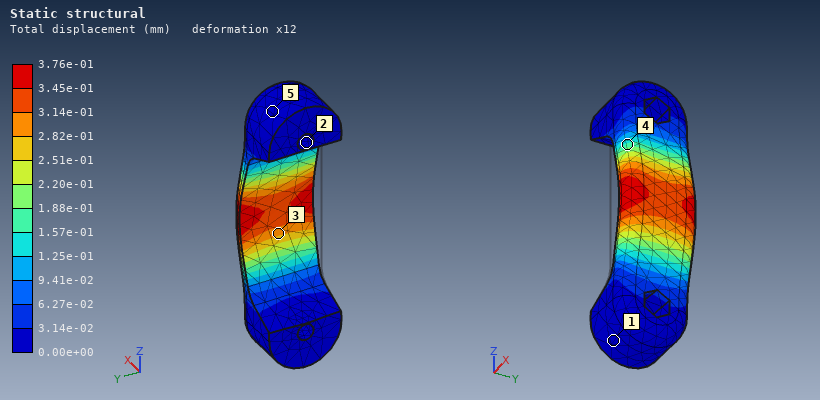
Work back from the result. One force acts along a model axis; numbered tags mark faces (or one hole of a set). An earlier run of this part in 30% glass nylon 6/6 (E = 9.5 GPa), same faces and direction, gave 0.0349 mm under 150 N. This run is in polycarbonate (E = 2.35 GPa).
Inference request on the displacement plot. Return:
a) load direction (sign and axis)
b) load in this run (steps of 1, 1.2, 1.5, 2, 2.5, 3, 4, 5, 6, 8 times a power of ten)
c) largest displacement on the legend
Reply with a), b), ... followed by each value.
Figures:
a) +X
b) 400 N
c) 3.76e-01 mm
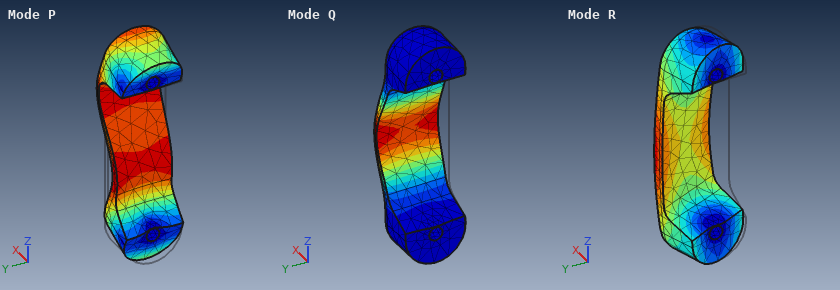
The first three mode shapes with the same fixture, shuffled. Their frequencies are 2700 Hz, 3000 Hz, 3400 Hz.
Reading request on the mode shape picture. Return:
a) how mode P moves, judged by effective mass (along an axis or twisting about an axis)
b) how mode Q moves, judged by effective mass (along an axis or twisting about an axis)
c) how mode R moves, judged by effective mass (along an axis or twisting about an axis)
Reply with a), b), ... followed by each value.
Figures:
a) along Z
b) along X
c) along Y
